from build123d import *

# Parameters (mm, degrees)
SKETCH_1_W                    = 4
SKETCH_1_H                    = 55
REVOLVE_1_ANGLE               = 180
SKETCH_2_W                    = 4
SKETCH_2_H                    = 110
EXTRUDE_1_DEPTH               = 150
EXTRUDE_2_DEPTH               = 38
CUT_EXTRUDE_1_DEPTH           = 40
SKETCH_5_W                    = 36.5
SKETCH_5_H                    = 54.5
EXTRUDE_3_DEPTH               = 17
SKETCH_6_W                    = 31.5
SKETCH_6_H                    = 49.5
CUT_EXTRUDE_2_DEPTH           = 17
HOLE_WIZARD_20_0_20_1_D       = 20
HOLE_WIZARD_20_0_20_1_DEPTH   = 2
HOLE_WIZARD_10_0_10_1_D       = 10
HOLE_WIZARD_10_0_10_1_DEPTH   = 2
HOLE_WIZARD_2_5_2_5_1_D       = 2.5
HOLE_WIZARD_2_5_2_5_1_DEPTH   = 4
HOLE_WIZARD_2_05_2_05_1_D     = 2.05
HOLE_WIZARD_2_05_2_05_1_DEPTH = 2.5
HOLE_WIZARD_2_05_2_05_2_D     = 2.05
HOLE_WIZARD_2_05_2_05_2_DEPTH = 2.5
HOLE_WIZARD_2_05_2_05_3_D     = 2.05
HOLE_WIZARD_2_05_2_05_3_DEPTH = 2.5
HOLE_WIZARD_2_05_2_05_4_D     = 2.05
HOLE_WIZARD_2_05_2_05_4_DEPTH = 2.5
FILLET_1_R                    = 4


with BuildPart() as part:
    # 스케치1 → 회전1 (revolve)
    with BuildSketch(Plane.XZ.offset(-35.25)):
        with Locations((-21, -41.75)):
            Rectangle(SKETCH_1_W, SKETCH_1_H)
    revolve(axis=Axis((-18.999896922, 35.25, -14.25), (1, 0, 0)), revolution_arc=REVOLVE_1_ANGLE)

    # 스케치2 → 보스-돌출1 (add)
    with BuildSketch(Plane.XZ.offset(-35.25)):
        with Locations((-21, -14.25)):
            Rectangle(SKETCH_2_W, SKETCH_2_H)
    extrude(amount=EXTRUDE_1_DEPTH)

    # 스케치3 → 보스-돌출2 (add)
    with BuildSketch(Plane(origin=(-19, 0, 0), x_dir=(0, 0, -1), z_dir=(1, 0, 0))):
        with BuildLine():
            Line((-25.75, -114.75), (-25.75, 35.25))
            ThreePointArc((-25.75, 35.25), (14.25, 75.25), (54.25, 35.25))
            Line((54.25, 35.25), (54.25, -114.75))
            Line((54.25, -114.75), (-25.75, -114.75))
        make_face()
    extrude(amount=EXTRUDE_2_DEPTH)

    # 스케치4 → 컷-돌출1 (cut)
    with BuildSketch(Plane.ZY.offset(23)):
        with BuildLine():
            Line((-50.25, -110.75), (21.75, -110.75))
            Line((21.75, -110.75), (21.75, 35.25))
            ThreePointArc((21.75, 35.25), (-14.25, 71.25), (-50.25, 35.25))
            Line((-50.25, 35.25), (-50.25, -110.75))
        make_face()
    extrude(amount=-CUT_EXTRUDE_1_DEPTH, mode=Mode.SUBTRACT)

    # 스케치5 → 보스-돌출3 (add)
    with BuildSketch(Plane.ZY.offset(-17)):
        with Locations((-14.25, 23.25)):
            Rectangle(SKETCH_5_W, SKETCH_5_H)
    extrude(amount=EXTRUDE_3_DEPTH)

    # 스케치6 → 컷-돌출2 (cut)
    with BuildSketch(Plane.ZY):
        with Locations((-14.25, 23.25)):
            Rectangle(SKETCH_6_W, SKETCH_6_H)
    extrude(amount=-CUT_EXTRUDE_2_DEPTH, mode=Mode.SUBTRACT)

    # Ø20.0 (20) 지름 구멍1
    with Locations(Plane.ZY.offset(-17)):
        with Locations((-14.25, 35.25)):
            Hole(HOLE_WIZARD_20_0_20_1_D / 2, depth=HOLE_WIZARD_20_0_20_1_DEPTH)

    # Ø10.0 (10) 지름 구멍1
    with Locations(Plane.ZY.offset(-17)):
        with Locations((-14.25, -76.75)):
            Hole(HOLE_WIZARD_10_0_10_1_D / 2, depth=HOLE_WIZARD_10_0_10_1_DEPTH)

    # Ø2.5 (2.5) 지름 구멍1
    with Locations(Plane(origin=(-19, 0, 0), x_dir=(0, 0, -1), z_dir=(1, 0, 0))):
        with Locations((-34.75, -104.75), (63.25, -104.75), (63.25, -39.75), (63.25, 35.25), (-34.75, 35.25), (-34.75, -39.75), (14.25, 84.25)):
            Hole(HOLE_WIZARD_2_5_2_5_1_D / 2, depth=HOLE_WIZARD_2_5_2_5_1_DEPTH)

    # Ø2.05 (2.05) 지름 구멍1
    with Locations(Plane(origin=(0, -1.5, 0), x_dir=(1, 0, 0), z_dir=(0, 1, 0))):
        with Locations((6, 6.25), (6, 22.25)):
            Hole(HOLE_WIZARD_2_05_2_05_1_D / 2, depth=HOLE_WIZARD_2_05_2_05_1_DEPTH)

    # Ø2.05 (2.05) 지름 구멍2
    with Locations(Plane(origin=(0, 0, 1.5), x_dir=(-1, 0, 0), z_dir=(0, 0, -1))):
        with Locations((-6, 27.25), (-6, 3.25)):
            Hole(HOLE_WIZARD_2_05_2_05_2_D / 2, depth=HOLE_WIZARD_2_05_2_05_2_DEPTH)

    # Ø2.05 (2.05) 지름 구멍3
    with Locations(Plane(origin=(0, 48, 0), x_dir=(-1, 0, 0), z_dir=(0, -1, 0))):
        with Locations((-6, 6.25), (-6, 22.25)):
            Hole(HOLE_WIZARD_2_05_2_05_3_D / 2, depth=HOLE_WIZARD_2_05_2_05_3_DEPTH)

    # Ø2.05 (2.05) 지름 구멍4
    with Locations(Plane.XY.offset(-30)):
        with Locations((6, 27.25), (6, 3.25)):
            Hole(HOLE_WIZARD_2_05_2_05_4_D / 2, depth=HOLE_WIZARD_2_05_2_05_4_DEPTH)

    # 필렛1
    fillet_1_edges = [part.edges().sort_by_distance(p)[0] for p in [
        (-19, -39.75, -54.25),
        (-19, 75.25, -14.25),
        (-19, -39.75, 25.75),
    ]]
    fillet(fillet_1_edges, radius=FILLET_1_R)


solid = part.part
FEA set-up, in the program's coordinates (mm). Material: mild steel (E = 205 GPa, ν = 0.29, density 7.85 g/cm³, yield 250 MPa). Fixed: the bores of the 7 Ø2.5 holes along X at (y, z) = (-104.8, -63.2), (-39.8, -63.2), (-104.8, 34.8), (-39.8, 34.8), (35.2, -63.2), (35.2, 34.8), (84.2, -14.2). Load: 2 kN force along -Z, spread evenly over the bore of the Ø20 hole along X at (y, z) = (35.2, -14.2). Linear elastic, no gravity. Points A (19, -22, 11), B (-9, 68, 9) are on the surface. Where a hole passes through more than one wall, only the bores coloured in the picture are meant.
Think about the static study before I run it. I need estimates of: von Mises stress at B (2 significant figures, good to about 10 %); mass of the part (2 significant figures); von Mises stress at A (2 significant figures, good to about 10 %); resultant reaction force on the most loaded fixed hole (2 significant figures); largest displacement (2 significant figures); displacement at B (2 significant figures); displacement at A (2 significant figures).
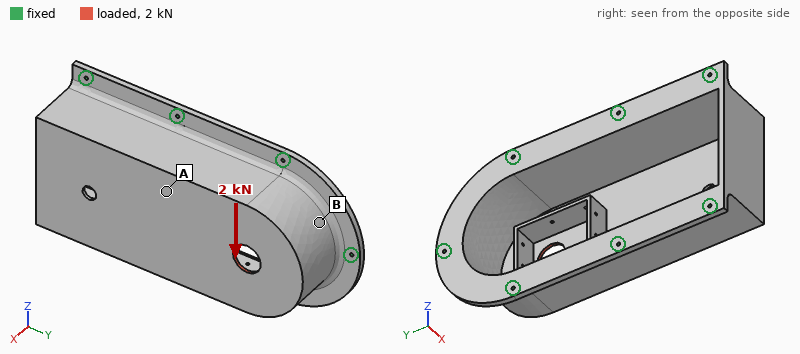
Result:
4.7 MPa
1.1 kg
9.9 MPa
750 N
17 µm
4.4 µm
13 µm
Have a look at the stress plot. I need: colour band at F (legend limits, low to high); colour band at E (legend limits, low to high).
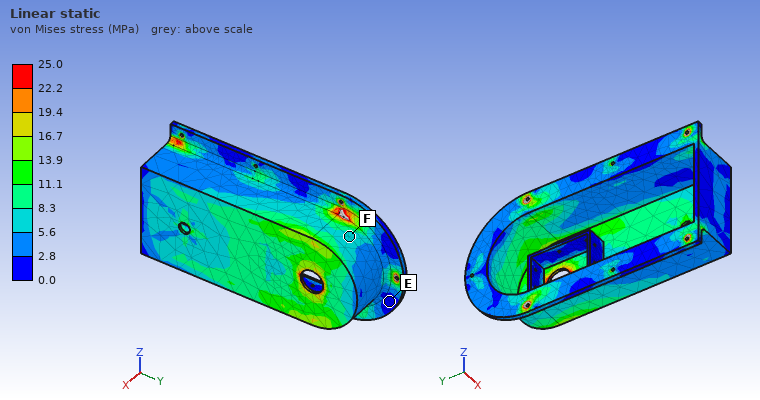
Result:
5.6 to 8.3 MPa
0.0 to 2.8 MPa
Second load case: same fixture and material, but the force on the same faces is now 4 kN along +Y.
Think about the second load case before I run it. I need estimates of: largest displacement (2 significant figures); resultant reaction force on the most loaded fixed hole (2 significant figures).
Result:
12 µm
800 N
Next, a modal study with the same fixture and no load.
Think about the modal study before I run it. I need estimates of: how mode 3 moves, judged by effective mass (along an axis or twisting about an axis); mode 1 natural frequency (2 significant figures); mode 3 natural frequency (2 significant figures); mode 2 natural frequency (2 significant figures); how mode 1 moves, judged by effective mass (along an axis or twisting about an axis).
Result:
along Z
2300 Hz
3000 Hz
2700 Hz
along X
